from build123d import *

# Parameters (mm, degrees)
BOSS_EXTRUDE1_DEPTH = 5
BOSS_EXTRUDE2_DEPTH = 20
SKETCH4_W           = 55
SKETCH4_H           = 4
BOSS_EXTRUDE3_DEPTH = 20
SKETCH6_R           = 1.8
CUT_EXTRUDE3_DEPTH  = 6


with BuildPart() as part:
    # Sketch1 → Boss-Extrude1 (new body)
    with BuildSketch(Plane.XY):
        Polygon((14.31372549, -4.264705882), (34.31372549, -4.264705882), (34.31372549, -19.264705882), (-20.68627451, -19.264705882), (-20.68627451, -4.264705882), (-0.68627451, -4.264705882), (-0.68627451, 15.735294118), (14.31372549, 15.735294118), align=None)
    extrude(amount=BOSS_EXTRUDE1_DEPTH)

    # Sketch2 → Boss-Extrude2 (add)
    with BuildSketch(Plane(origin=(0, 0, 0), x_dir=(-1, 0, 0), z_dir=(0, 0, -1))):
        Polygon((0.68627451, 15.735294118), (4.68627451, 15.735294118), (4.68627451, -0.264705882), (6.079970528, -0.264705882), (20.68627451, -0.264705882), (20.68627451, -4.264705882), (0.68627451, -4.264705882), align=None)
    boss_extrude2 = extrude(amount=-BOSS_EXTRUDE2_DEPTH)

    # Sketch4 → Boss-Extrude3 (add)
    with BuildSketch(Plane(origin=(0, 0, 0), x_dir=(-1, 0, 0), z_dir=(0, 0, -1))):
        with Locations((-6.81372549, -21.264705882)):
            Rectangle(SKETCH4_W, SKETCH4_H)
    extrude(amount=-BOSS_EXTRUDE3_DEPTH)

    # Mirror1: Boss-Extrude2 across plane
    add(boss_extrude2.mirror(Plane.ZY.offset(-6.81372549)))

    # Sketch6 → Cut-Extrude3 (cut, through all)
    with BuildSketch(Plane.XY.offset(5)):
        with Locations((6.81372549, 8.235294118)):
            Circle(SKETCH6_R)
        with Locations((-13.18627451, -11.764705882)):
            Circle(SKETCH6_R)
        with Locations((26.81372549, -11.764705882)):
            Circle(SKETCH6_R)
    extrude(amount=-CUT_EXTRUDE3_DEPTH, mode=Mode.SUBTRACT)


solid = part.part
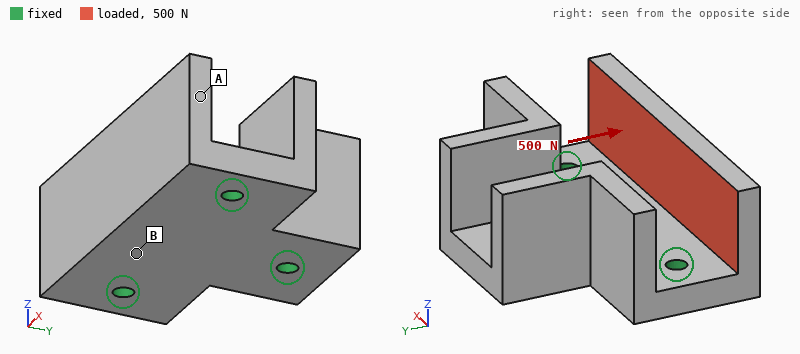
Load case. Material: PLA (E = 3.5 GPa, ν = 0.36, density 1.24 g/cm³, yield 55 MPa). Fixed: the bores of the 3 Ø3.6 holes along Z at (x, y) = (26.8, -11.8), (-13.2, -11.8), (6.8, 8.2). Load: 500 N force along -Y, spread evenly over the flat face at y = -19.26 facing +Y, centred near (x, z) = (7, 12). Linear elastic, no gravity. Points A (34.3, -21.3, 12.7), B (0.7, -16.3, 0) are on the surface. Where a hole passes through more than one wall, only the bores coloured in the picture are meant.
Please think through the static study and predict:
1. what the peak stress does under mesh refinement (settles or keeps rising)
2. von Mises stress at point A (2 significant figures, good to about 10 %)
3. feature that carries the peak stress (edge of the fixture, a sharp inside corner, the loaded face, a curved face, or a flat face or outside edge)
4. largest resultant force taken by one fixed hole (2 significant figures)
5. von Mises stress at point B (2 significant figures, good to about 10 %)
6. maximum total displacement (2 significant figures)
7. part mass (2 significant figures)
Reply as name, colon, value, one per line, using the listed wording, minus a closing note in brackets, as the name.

what the peak stress does under mesh refinement: keeps rising
von Mises stress at point A: 4.2 MPa
feature that carries the peak stress: edge of the fixture
largest resultant force taken by one fixed hole: 190 N
von Mises stress at point B: 15 MPa
maximum total displacement: 0.75 mm
part mass: 19 g
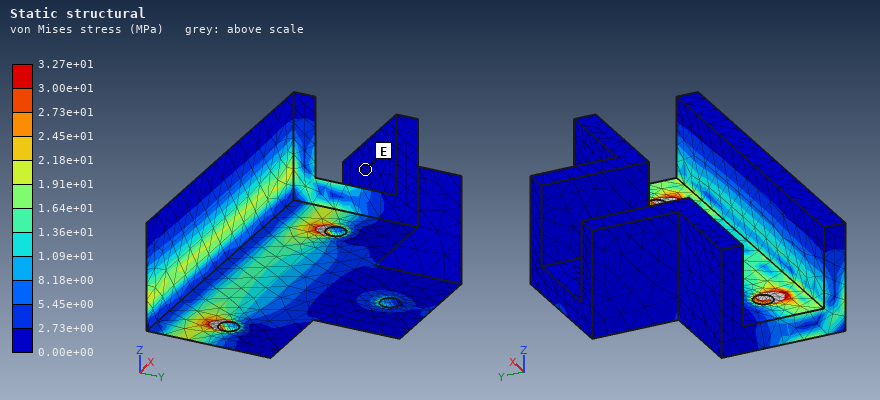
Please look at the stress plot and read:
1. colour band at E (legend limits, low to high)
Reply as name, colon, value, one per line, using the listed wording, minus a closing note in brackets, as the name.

colour band at E: 0.00e+00 to 2.73e+00 MPa
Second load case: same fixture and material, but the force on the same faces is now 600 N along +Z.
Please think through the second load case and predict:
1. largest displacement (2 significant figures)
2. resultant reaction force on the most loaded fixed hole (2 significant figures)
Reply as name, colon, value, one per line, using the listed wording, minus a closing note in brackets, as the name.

largest displacement: 0.18 mm
resultant reaction force on the most loaded fixed hole: 320 N
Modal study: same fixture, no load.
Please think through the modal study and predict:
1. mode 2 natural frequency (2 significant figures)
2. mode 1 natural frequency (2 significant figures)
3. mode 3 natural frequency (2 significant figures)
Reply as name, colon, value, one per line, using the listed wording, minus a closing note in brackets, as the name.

mode 2 natural frequency: 3200 Hz
mode 1 natural frequency: 2300 Hz
mode 3 natural frequency: 3400 Hz
